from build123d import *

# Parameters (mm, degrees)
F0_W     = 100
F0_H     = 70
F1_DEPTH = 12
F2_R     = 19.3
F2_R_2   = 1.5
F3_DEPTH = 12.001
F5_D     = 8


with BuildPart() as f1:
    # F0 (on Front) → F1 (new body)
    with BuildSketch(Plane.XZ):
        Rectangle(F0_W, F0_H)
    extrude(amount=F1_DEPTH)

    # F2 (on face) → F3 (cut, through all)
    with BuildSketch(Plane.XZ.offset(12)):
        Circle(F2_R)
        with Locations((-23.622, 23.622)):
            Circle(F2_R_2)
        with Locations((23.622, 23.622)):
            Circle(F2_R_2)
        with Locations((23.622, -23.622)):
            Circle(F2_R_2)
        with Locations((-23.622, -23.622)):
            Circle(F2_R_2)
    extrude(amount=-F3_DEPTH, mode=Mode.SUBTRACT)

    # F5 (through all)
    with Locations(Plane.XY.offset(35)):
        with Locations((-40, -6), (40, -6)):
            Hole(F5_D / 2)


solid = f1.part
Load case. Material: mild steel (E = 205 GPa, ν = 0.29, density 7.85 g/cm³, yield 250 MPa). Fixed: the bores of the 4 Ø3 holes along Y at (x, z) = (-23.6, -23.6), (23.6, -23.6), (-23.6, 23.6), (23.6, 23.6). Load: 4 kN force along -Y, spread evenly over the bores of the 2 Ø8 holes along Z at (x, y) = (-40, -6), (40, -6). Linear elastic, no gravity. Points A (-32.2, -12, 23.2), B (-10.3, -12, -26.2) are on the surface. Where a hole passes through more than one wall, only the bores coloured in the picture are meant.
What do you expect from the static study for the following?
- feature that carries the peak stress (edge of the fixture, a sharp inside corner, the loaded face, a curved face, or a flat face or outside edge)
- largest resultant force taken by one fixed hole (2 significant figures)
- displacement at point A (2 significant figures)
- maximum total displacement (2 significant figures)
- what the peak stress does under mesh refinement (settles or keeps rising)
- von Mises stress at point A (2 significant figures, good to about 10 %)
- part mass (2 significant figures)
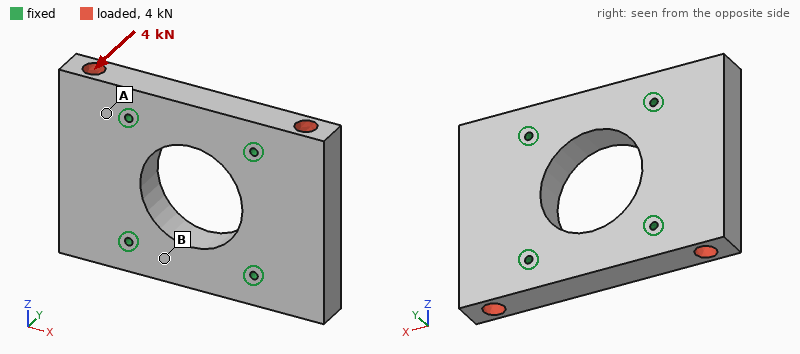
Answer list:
edge of the fixture
1.0 kN
2.4 µm
9.5 µm
keeps rising
15 MPa
490 g
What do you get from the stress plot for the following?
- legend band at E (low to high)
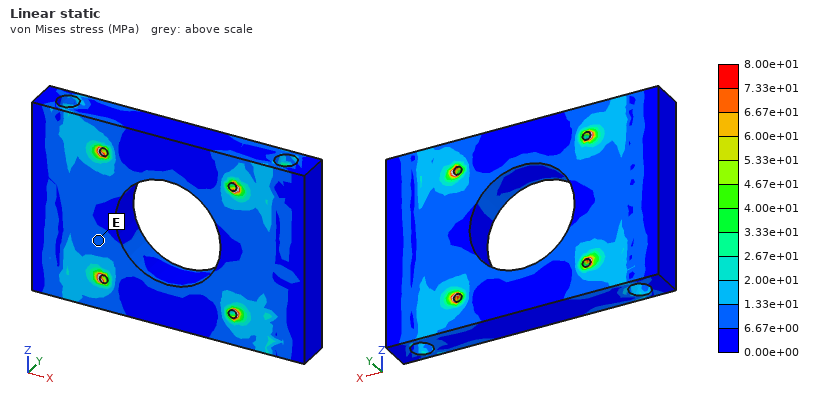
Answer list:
6.67e+00 to 1.33e+01 MPa
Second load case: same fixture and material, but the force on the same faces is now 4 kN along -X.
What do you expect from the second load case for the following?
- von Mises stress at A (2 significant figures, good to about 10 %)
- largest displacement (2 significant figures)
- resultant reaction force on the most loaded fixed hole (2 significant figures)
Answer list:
5.5 MPa
0.72 µm
1.0 kN
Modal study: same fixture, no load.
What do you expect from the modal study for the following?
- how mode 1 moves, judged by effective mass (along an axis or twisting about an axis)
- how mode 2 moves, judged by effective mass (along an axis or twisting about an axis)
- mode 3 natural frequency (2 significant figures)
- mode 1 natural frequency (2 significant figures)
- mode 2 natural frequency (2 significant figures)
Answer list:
along Y
twisting about Z
13 kHz
8300 Hz
8700 Hz
